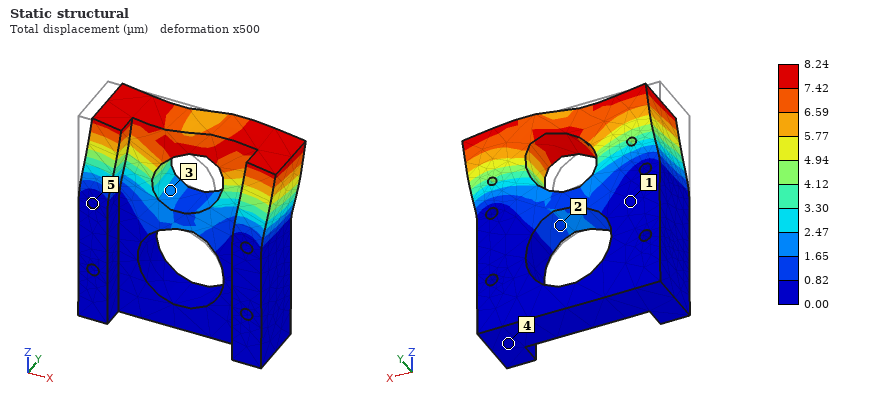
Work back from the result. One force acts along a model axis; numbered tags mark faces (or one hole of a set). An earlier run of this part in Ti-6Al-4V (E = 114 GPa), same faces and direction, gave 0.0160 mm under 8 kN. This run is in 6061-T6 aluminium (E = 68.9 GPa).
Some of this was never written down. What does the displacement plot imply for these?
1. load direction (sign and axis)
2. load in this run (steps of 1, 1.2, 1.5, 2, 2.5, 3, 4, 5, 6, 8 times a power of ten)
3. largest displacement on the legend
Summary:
+X
2.5 kN
8.24 µm
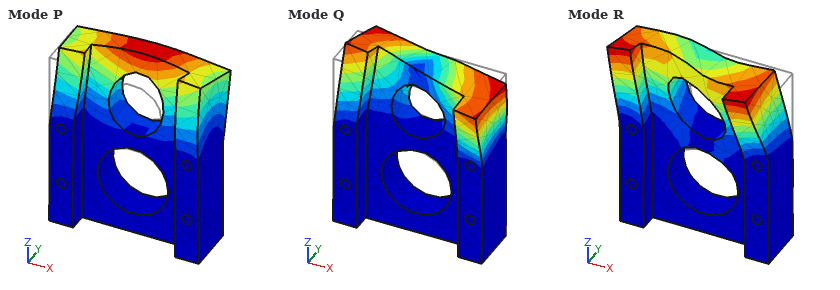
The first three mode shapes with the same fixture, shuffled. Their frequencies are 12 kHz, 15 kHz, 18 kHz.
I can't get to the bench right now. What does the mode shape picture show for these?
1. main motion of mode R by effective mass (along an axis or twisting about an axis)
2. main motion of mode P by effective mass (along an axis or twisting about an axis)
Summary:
along X
along Y
